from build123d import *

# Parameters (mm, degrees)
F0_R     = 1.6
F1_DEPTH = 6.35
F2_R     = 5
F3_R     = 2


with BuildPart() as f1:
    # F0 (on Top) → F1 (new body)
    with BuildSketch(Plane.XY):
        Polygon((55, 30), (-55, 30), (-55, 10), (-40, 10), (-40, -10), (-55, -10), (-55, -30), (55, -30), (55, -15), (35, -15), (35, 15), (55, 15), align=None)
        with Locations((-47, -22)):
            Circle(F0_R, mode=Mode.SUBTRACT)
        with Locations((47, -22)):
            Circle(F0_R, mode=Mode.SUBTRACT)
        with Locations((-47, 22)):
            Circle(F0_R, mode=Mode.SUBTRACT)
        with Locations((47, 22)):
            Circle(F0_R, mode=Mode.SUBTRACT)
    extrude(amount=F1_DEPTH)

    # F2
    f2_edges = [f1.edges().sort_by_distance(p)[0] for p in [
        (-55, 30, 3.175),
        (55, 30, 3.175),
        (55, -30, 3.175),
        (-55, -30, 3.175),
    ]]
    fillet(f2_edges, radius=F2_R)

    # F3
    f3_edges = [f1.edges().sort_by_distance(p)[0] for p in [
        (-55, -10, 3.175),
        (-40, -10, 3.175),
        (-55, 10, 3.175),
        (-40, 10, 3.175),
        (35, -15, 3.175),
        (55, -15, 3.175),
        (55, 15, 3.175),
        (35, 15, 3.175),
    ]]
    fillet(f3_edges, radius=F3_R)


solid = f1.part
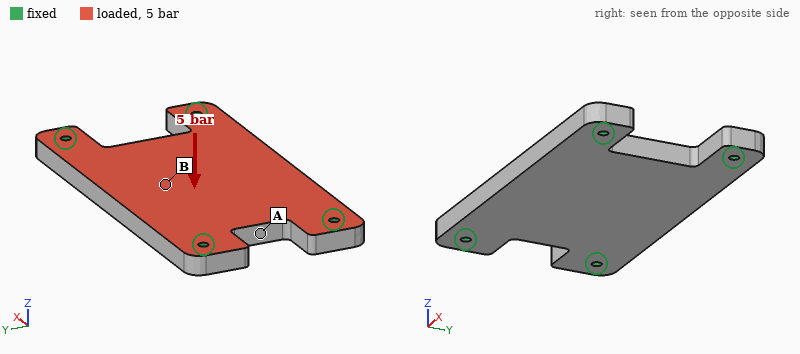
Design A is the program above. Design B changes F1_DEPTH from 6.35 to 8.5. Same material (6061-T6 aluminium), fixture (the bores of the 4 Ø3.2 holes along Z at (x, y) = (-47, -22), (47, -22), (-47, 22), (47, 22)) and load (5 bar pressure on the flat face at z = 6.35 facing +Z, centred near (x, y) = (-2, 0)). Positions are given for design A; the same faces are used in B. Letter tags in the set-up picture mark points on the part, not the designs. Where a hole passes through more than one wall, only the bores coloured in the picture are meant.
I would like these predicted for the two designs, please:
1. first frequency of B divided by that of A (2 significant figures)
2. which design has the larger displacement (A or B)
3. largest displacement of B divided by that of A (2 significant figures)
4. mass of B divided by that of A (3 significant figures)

1.3
A
0.45
1.34
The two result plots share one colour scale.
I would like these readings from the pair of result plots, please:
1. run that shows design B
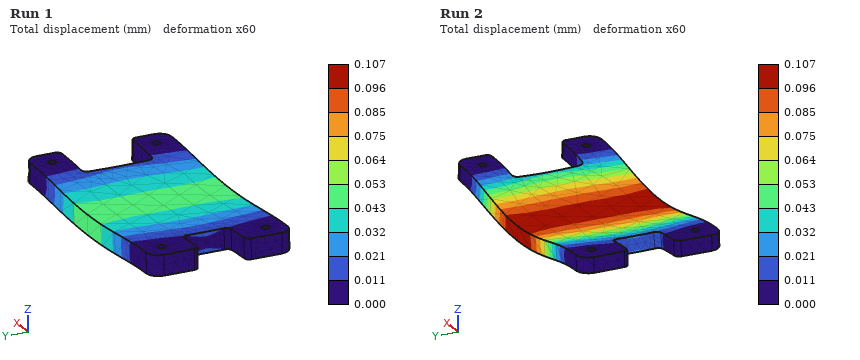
Run 1
